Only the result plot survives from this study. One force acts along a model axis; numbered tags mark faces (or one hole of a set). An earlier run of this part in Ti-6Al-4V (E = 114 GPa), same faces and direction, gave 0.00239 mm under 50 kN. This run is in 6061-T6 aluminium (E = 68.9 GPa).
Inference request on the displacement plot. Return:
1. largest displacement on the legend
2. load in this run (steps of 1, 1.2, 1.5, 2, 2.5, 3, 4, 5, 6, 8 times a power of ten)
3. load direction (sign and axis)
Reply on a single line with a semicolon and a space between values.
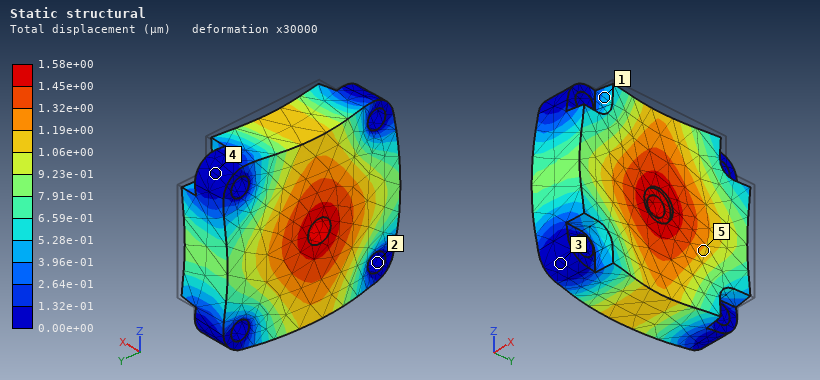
1.58e+00 µm; 20 kN; -X
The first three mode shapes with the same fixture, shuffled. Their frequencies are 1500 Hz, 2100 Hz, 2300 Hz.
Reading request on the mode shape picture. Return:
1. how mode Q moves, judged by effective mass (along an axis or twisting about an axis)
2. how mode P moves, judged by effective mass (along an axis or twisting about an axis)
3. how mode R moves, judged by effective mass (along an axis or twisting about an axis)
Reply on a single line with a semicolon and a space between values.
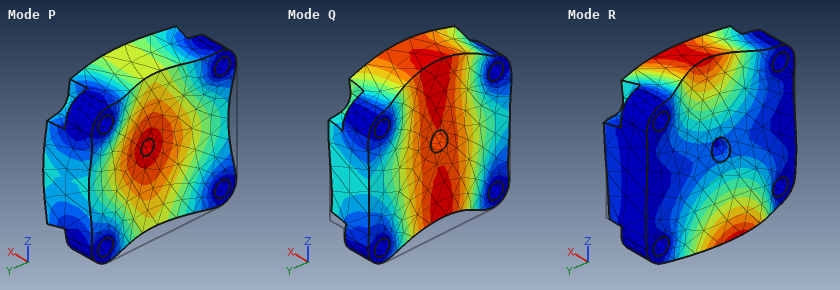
along Z; along X; twisting about Y
